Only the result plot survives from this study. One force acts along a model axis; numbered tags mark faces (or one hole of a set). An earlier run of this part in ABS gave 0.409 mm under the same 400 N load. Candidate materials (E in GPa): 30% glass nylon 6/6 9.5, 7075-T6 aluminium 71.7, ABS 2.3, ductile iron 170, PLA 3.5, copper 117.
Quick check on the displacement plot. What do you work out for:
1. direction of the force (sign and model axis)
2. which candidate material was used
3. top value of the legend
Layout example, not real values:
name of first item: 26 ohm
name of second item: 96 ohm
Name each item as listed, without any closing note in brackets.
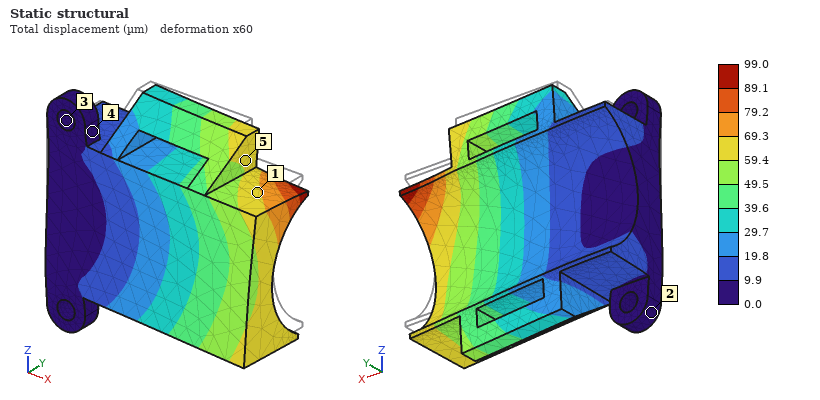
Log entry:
direction of the force: -Z
which candidate material was used: 30% glass nylon 6/6
top value of the legend: 99.0 µm
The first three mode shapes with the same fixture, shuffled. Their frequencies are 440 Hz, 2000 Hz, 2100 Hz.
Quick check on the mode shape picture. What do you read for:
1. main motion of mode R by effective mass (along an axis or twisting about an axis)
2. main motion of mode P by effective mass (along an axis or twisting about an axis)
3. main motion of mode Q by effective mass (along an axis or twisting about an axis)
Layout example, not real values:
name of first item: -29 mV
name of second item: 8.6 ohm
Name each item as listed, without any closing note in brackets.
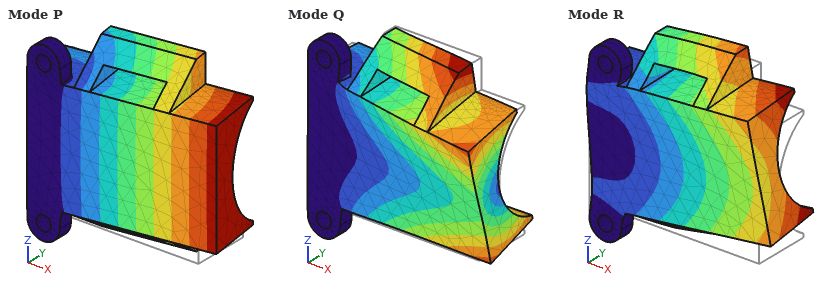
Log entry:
main motion of mode R by effective mass: along Z
main motion of mode P by effective mass: along Y
main motion of mode Q by effective mass: twisting about X
